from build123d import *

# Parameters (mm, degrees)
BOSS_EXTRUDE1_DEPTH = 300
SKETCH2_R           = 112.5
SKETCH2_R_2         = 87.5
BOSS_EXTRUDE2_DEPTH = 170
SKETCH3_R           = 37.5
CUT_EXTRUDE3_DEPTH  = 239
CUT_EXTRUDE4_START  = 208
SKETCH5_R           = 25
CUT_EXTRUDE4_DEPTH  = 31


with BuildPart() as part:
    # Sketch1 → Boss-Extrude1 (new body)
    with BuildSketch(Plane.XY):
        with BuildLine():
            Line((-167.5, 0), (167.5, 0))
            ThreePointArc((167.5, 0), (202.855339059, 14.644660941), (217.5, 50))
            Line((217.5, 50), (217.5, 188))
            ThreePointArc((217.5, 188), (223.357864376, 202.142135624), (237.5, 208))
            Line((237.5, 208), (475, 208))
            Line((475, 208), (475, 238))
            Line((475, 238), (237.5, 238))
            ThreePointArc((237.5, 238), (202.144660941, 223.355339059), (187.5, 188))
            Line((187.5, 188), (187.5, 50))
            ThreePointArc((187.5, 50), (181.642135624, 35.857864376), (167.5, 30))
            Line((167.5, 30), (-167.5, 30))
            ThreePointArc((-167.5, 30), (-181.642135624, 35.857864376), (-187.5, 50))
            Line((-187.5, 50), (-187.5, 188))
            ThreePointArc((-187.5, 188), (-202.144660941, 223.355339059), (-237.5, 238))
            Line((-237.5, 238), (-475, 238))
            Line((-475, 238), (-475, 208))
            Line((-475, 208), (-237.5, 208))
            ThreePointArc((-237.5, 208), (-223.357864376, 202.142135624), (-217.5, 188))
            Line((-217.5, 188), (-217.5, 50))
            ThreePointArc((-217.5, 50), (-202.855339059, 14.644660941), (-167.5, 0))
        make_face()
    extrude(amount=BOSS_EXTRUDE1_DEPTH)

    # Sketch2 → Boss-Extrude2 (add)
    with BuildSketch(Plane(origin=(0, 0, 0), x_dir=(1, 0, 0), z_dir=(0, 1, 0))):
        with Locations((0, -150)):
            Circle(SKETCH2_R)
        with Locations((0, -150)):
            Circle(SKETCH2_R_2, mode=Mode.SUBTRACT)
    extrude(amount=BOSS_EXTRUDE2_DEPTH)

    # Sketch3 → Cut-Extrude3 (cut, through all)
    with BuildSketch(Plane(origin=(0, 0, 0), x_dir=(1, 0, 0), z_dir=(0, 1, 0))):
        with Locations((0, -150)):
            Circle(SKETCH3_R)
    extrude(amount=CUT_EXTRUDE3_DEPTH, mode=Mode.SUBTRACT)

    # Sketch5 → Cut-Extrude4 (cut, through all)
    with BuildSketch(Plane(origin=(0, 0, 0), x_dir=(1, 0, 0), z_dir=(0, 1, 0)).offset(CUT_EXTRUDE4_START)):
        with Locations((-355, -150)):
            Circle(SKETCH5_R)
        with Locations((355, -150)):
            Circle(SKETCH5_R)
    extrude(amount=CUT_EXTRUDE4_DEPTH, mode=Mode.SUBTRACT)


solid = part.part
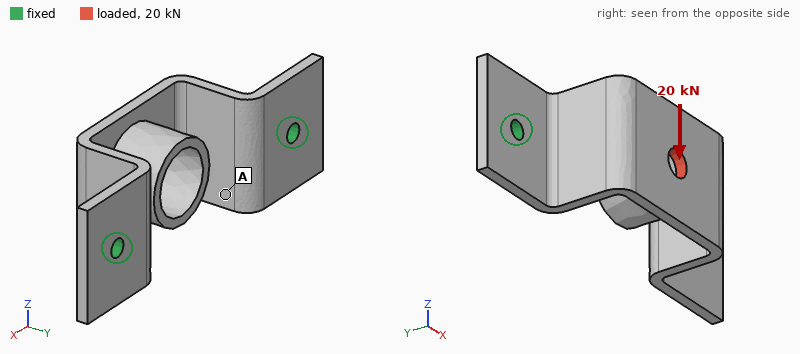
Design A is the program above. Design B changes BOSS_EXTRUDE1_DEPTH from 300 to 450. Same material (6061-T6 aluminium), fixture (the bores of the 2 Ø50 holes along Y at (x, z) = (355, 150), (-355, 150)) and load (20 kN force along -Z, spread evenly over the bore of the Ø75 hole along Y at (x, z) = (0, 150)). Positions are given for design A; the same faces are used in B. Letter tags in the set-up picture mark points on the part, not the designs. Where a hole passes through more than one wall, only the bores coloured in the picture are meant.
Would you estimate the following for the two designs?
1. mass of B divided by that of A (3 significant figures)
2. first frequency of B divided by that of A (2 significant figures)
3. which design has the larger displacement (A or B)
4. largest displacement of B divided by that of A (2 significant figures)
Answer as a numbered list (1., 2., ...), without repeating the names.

1. 1.43
2. 0.75
3. B
4. 1.1
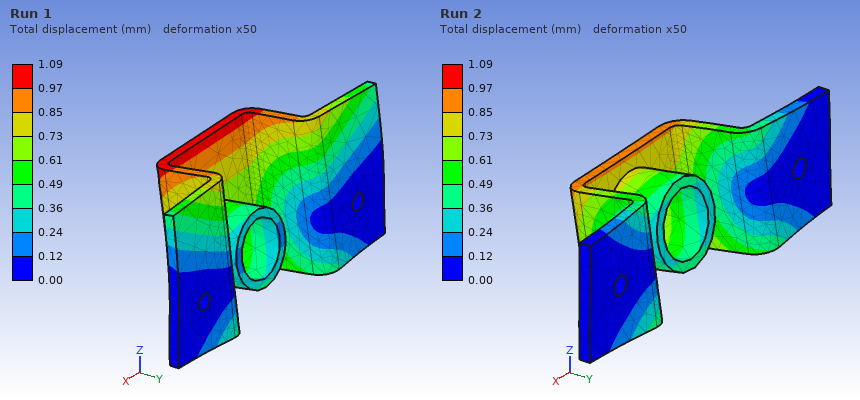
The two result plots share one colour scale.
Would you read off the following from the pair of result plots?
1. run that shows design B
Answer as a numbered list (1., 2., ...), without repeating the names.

1. Run 1
